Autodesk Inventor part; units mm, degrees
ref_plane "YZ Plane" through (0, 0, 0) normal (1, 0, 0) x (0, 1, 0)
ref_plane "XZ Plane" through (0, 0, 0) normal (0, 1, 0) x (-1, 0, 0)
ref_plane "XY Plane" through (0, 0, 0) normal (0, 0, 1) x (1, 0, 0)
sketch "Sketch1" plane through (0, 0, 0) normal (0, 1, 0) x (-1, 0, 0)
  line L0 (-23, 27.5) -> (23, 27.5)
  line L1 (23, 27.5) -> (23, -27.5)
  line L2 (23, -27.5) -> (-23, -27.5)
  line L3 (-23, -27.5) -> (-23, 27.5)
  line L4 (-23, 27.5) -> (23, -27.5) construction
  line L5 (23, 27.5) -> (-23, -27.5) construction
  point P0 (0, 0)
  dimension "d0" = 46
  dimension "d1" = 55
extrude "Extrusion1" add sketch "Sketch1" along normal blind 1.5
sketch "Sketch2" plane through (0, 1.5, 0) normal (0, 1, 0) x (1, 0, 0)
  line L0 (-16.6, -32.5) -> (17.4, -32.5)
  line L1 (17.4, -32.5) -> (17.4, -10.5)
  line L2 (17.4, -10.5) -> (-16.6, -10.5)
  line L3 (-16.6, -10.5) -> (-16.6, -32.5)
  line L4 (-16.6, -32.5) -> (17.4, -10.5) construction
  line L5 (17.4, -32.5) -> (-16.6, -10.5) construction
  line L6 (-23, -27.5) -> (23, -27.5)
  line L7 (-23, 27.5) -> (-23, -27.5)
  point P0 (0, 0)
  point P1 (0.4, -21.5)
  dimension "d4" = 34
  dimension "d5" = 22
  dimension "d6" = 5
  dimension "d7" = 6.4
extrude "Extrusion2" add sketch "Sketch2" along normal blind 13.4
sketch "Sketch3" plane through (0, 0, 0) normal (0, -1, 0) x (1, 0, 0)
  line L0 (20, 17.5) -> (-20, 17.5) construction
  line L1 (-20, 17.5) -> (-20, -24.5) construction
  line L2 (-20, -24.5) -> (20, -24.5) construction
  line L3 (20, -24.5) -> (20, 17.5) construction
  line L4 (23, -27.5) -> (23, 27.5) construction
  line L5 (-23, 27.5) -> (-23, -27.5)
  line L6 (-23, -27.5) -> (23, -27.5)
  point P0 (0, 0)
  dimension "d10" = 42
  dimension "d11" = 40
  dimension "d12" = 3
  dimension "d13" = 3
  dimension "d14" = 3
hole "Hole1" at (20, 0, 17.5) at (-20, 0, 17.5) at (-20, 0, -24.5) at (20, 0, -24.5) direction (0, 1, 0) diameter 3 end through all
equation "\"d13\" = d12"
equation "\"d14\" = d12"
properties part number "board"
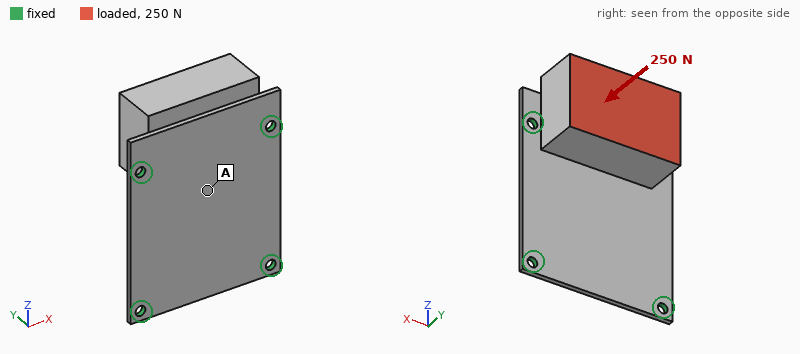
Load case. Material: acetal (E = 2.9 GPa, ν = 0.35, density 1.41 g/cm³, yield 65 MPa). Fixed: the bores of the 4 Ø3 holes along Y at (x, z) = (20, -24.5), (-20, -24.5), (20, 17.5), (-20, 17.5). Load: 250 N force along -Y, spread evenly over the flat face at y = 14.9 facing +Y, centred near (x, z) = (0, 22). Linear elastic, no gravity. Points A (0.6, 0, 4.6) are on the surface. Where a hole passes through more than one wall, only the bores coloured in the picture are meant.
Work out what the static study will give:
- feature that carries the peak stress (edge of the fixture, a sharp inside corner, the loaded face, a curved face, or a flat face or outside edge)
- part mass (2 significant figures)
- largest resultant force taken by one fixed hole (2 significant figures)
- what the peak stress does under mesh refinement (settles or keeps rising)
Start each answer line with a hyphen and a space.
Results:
- edge of the fixture
- 19 g
- 150 N
- keeps rising
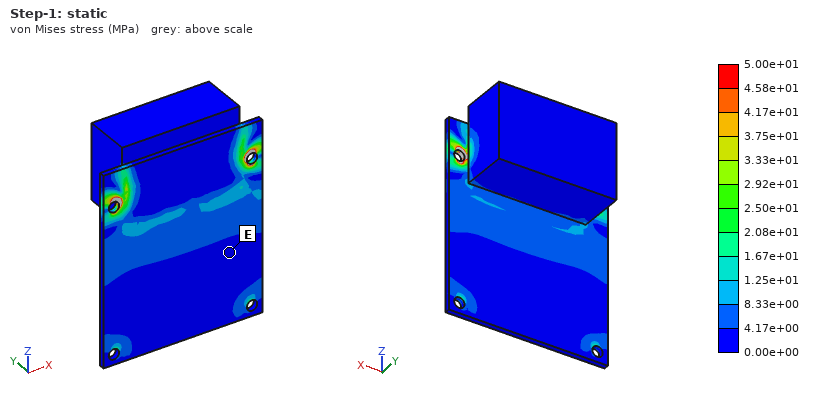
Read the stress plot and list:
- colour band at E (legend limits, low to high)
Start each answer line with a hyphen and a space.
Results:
- 0.00e+00 to 4.17e+00 MPa
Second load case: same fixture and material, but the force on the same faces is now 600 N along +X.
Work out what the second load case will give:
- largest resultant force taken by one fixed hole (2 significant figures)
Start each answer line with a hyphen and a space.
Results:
- 380 N
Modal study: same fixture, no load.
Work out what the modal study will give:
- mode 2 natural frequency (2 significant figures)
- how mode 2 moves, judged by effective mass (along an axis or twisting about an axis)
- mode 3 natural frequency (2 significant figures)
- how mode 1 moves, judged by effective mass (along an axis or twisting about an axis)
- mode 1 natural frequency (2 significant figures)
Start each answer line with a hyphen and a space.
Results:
- 1300 Hz
- along Y
- 1800 Hz
- along Z
- 570 Hz
